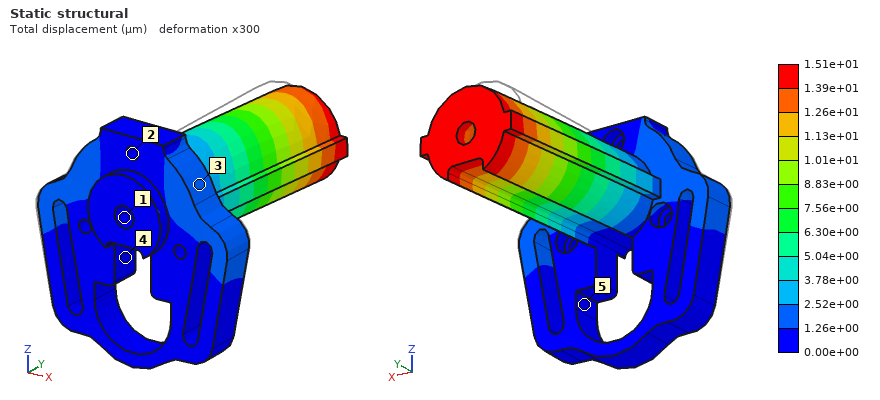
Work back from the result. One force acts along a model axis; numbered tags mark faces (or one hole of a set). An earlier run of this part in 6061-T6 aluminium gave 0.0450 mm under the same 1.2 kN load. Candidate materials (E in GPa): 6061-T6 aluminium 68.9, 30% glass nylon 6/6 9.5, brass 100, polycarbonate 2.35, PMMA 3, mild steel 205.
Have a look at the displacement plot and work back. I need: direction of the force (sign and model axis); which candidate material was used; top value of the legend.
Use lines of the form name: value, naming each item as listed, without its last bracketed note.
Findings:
direction of the force: +X
which candidate material was used: mild steel
top value of the legend: 1.51e+01 µm
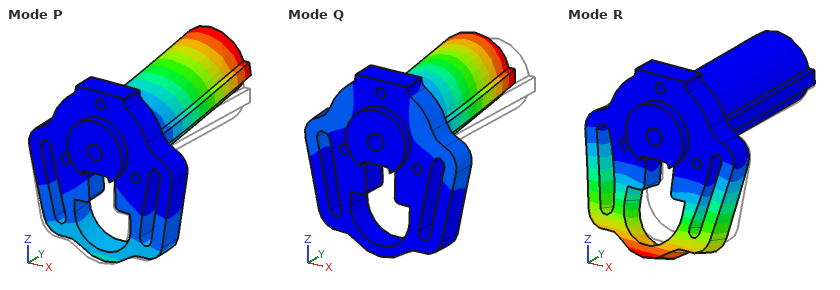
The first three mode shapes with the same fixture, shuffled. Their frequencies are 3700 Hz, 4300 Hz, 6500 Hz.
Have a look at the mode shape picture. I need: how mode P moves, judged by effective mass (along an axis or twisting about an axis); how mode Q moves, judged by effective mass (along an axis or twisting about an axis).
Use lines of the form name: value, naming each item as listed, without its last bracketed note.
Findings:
how mode P moves, judged by effective mass: along Z
how mode Q moves, judged by effective mass: along X
